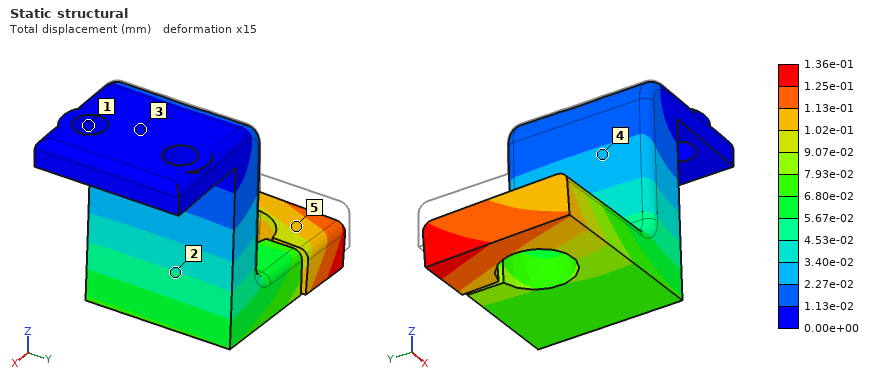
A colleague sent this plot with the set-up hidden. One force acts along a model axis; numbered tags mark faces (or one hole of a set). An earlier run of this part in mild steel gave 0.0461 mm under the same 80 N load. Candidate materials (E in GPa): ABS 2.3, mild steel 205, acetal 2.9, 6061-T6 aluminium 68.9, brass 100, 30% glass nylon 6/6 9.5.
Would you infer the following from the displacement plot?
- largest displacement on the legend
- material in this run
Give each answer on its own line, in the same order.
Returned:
1.36e-01 mm
6061-T6 aluminium
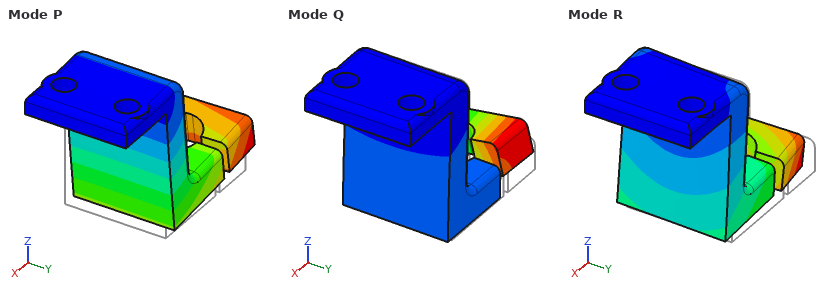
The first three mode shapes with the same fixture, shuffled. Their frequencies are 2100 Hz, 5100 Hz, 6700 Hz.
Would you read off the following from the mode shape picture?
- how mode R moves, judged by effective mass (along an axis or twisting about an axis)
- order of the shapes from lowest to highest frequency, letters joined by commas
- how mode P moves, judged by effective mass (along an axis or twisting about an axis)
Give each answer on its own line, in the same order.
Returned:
along Y
P, R, Q
along X
